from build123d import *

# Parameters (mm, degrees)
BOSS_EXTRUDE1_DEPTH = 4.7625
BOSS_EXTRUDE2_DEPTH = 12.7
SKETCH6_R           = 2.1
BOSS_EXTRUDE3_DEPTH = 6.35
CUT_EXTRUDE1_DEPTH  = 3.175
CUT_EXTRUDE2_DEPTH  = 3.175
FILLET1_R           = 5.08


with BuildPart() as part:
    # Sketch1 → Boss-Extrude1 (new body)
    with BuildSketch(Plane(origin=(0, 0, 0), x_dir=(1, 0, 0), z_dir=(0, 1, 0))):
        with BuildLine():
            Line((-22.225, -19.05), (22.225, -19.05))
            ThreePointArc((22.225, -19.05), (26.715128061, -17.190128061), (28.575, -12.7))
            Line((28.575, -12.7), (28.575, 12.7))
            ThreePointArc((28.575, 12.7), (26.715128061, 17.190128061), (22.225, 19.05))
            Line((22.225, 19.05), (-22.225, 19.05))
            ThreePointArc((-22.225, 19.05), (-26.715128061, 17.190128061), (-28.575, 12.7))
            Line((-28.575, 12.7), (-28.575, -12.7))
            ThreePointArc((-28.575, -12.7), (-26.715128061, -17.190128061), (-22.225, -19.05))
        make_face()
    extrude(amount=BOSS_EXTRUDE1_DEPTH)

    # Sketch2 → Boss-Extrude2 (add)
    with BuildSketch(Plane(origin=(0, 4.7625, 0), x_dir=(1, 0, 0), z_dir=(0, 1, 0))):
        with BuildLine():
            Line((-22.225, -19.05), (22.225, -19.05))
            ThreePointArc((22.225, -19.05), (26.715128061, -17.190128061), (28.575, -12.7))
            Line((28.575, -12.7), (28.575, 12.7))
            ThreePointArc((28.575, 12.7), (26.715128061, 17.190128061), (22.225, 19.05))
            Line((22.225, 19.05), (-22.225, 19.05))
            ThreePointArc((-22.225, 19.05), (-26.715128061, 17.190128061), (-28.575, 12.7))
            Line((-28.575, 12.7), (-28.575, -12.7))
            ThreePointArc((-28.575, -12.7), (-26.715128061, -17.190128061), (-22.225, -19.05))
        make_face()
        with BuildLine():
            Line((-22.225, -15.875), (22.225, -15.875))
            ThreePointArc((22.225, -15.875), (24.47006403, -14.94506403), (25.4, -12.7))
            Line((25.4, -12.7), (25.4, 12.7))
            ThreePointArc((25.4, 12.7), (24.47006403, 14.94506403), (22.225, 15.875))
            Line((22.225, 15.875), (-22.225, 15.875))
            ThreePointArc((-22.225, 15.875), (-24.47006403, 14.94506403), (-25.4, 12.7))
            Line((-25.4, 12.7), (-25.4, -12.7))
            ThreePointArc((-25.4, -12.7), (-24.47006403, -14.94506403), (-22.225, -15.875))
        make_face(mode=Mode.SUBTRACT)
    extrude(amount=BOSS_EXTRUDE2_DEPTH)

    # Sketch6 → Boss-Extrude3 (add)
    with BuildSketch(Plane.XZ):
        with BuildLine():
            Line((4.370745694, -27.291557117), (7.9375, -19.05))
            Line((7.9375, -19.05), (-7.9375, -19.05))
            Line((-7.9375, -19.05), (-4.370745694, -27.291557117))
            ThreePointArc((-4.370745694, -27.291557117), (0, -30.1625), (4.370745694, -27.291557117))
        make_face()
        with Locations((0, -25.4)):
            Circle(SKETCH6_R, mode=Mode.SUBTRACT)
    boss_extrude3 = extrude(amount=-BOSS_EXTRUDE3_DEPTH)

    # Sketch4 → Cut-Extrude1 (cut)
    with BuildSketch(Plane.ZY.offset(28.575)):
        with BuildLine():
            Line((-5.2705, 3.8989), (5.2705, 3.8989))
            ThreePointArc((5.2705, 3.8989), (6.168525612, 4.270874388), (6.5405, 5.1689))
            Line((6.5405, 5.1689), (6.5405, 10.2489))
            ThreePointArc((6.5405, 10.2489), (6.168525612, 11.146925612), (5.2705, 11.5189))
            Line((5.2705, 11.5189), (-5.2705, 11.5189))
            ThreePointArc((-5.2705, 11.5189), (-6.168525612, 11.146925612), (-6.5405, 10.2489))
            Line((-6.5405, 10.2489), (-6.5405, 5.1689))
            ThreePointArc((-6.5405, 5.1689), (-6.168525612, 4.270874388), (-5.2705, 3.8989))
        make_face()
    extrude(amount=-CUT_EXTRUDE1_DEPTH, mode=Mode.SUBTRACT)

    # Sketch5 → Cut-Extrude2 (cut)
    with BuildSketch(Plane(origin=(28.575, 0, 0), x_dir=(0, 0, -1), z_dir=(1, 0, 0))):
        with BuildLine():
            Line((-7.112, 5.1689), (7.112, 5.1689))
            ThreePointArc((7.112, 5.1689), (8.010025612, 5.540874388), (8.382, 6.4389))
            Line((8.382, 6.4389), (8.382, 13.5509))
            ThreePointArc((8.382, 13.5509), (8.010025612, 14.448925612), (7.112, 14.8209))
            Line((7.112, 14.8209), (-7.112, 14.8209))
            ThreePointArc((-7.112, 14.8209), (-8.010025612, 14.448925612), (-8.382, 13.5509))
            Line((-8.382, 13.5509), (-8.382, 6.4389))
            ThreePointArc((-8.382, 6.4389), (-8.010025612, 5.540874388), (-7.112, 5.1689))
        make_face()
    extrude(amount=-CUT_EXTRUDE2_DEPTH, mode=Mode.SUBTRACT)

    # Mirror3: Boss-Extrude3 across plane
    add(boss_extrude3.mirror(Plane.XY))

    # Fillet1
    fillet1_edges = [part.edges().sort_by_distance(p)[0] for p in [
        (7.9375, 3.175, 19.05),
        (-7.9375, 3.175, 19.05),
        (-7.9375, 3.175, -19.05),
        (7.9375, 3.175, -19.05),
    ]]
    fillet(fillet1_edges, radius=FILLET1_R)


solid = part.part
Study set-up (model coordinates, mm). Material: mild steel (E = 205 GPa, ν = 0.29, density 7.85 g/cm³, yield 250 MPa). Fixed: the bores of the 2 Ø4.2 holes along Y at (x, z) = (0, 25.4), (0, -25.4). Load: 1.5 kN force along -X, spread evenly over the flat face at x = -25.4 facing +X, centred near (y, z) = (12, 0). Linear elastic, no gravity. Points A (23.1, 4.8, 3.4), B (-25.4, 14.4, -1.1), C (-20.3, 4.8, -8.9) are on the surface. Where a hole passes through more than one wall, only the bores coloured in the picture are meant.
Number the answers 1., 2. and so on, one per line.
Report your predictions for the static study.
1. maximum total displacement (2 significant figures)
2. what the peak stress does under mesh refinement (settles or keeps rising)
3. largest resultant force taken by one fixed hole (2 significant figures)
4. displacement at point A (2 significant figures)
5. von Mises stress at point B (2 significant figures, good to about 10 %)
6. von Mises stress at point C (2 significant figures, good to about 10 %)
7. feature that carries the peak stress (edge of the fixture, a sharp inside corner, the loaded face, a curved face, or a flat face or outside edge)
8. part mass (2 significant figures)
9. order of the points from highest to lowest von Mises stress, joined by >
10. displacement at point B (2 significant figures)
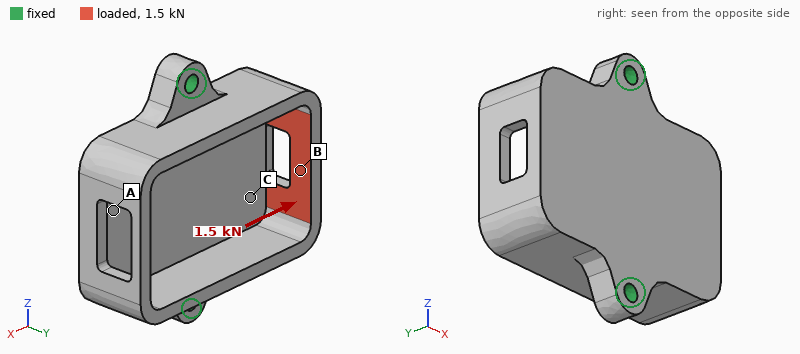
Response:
1. 62 µm
2. keeps rising
3. 760 N
4. 16 µm
5. 130 MPa
6. 27 MPa
7. a sharp inside corner
8. 140 g
9. B > C > A
10. 49 µm
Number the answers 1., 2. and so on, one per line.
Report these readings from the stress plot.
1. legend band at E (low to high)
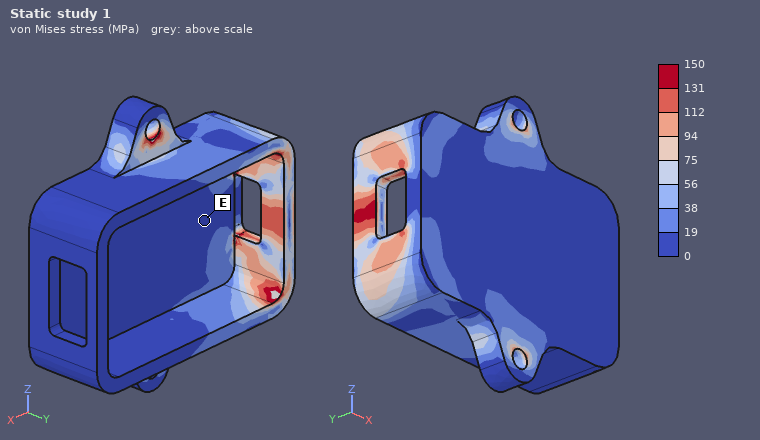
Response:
1. 0 to 19 MPa
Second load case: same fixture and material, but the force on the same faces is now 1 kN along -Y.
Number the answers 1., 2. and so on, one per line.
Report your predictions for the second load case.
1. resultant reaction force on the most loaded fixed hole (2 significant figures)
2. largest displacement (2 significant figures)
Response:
1. 500 N
2. 54 µm
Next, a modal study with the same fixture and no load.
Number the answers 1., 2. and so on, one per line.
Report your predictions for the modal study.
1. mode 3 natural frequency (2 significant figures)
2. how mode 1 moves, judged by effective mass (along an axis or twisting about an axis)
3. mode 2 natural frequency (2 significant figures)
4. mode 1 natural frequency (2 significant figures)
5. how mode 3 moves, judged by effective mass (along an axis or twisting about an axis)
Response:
1. 7100 Hz
2. twisting about Z
3. 6600 Hz
4. 3300 Hz
5. along Y
